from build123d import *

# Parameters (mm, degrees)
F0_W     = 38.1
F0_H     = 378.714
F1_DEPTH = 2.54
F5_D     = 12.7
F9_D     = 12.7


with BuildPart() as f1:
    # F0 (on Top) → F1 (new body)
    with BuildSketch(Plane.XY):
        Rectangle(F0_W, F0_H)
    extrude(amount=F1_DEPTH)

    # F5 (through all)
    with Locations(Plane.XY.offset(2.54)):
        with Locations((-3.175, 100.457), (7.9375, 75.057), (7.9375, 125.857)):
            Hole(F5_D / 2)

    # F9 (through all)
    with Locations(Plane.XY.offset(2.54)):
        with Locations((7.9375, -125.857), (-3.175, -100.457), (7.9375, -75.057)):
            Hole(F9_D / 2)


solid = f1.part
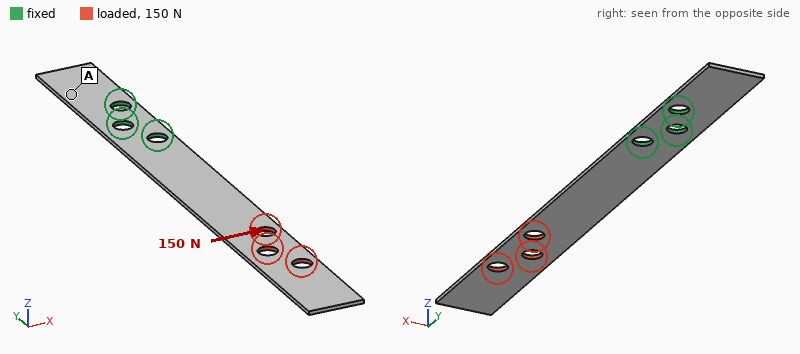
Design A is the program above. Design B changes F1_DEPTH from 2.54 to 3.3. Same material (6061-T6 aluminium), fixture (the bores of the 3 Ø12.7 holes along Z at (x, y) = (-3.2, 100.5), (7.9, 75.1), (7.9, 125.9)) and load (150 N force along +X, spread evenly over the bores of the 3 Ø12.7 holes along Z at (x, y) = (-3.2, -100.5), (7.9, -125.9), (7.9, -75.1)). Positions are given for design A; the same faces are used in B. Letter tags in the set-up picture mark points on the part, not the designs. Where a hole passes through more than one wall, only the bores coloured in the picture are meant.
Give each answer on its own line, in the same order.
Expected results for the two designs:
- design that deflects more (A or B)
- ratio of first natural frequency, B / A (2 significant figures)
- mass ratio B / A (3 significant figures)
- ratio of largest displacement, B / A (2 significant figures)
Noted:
A
1.3
1.30
0.77
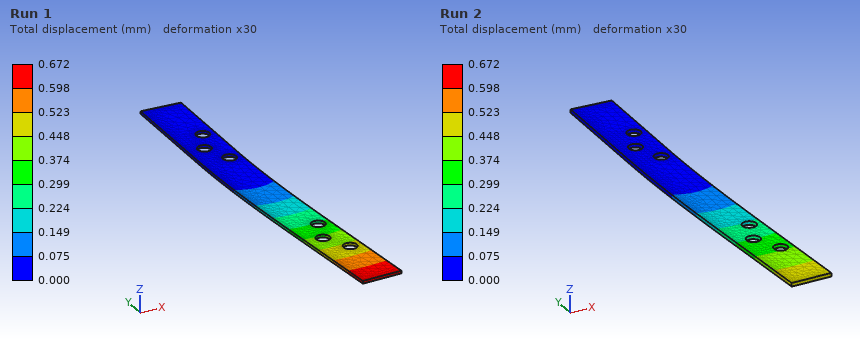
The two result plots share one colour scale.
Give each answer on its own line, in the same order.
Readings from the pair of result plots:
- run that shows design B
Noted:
Run 2
